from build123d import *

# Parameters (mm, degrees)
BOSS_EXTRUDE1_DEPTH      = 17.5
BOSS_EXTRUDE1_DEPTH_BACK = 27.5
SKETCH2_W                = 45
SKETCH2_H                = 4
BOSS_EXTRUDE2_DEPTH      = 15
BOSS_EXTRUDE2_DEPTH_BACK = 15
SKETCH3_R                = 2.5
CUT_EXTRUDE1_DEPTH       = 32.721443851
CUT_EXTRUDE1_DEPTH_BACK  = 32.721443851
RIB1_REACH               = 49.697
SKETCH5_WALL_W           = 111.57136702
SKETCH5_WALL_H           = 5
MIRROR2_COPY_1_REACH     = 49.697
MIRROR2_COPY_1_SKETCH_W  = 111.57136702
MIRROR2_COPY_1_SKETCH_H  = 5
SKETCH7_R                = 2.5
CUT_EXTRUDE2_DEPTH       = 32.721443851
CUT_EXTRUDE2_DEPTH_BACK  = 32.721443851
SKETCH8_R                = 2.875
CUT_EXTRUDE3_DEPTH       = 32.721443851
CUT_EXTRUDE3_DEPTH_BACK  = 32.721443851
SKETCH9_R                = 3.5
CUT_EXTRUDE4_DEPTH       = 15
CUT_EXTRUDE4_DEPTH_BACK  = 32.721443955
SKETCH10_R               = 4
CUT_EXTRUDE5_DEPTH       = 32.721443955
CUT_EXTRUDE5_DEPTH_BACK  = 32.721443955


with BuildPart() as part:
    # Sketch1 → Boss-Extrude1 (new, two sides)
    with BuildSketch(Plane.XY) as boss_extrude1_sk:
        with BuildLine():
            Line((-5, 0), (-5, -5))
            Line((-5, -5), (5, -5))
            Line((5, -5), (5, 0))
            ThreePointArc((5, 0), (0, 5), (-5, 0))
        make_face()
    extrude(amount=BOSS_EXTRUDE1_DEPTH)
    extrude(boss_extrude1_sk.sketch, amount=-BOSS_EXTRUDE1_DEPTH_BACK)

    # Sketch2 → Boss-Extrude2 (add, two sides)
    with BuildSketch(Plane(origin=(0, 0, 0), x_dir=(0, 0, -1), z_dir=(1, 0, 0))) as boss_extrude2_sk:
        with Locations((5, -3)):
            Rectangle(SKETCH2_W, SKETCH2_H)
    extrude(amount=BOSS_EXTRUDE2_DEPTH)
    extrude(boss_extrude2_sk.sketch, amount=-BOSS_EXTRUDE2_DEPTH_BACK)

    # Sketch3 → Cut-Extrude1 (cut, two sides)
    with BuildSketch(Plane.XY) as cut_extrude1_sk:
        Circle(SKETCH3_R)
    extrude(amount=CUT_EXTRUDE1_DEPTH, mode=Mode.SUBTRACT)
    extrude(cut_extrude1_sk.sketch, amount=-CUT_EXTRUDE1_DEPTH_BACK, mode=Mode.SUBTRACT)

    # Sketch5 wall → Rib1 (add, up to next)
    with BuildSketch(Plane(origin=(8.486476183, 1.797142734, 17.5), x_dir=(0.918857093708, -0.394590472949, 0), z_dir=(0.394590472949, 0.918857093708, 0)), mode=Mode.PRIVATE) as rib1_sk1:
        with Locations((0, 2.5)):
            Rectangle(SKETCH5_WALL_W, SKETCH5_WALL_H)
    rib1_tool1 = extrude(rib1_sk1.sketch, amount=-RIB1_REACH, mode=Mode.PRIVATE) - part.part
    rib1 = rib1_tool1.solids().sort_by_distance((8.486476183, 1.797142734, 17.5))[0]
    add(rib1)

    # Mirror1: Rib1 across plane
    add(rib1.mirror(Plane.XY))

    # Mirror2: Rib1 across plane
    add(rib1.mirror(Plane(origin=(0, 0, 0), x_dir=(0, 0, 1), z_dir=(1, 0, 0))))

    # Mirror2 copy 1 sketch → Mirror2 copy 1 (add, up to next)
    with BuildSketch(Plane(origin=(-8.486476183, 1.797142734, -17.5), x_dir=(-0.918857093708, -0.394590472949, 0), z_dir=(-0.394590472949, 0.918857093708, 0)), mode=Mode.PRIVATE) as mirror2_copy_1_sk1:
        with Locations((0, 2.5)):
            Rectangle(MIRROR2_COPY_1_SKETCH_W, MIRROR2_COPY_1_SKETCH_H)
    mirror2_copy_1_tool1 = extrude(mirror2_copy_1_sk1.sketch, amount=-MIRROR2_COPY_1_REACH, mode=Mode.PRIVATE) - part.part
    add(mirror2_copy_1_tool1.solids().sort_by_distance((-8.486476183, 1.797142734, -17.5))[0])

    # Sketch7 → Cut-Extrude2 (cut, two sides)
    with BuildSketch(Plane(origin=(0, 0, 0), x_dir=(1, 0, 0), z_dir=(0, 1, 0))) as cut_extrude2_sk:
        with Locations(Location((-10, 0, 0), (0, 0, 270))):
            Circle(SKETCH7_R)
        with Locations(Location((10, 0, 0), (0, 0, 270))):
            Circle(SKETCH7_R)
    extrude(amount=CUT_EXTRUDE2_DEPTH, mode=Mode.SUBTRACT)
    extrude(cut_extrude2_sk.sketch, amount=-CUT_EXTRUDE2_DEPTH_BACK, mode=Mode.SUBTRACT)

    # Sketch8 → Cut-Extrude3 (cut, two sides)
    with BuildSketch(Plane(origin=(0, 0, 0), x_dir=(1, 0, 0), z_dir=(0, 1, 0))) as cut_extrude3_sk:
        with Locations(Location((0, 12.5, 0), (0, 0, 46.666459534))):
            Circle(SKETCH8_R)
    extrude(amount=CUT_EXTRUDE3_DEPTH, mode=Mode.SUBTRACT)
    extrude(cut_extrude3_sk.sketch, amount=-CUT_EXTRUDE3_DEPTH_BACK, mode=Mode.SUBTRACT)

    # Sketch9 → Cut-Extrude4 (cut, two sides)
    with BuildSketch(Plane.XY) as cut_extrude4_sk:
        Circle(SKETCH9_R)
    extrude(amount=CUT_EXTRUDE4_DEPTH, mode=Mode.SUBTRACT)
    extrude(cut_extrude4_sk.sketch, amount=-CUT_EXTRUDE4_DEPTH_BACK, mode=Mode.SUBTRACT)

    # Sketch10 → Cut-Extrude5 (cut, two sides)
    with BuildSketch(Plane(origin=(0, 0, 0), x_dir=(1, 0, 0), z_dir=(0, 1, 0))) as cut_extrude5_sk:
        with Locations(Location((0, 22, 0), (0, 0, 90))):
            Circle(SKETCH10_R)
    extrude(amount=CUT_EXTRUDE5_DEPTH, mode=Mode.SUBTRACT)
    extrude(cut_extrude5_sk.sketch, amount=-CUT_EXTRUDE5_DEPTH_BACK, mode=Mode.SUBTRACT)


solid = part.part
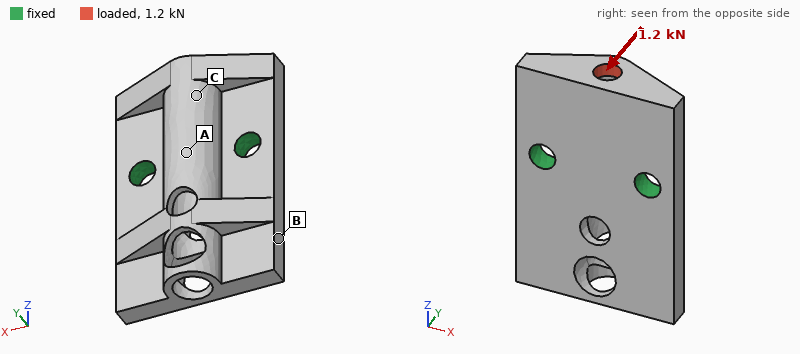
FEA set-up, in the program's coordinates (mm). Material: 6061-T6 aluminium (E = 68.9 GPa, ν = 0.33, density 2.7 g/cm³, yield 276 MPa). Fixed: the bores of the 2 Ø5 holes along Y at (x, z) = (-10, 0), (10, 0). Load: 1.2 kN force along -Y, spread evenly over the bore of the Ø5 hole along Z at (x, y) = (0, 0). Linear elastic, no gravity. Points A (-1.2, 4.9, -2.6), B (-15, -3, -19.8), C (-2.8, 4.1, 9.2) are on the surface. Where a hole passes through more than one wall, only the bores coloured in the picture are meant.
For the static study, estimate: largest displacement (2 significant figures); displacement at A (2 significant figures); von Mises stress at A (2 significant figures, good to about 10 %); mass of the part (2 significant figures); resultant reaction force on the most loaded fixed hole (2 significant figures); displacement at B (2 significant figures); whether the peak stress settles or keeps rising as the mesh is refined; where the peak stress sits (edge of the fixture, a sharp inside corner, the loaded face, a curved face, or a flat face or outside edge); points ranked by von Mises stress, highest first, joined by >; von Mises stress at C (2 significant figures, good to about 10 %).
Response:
100 µm
24 µm
44 MPa
16 g
630 N
41 µm
keeps rising
edge of the fixture
C > A > B
67 MPa
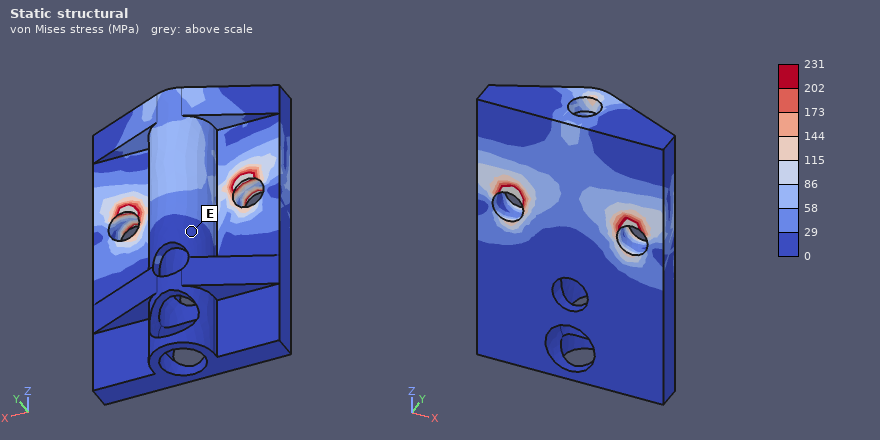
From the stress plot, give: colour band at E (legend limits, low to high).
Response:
0 to 29 MPa
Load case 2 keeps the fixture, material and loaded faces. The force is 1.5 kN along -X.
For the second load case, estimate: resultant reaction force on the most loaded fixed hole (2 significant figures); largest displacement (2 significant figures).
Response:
1.3 kN
20 µm
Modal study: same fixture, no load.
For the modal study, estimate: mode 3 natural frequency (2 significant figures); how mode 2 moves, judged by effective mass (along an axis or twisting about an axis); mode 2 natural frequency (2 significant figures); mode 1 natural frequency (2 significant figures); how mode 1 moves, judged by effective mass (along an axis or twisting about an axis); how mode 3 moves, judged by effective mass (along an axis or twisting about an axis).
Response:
13 kHz
twisting about Z
11 kHz
6000 Hz
along Y
along Y
